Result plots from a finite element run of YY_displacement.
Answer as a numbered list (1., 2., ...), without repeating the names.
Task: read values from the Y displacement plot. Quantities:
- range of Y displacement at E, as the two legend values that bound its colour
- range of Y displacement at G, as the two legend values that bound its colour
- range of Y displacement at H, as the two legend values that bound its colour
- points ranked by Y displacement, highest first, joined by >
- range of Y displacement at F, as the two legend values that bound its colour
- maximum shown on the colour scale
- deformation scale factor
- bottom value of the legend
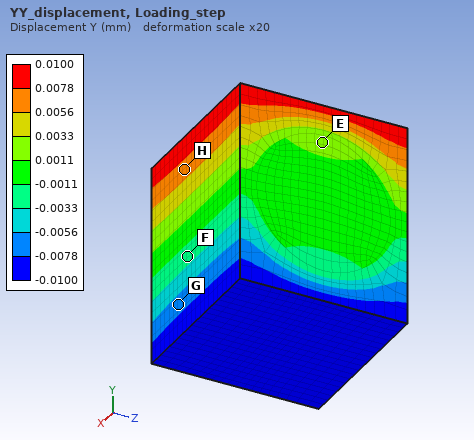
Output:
1. 0.0011 to 0.0033 mm
2. -0.0078 to -0.0056 mm
3. 0.0056 to 0.0078 mm
4. H > E > F > G
5. -0.0033 to -0.0011 mm
6. 0.0100 mm
7. 20
8. -0.0100 mm
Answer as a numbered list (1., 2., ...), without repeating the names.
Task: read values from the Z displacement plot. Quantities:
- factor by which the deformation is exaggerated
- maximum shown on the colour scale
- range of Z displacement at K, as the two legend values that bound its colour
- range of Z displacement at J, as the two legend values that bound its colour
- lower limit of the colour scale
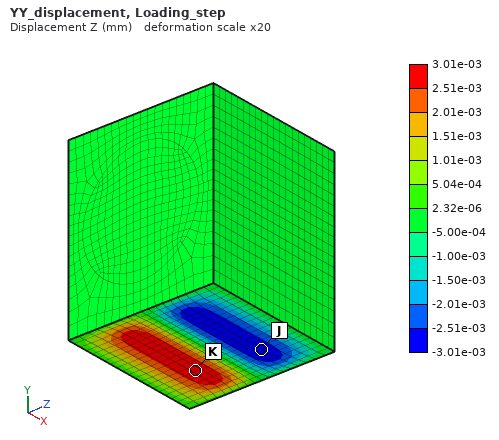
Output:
1. 20
2. 3.01e-03 mm
3. 2.51e-03 to 3.01e-03 mm
4. -3.01e-03 to -2.51e-03 mm
5. -3.01e-03 mm
